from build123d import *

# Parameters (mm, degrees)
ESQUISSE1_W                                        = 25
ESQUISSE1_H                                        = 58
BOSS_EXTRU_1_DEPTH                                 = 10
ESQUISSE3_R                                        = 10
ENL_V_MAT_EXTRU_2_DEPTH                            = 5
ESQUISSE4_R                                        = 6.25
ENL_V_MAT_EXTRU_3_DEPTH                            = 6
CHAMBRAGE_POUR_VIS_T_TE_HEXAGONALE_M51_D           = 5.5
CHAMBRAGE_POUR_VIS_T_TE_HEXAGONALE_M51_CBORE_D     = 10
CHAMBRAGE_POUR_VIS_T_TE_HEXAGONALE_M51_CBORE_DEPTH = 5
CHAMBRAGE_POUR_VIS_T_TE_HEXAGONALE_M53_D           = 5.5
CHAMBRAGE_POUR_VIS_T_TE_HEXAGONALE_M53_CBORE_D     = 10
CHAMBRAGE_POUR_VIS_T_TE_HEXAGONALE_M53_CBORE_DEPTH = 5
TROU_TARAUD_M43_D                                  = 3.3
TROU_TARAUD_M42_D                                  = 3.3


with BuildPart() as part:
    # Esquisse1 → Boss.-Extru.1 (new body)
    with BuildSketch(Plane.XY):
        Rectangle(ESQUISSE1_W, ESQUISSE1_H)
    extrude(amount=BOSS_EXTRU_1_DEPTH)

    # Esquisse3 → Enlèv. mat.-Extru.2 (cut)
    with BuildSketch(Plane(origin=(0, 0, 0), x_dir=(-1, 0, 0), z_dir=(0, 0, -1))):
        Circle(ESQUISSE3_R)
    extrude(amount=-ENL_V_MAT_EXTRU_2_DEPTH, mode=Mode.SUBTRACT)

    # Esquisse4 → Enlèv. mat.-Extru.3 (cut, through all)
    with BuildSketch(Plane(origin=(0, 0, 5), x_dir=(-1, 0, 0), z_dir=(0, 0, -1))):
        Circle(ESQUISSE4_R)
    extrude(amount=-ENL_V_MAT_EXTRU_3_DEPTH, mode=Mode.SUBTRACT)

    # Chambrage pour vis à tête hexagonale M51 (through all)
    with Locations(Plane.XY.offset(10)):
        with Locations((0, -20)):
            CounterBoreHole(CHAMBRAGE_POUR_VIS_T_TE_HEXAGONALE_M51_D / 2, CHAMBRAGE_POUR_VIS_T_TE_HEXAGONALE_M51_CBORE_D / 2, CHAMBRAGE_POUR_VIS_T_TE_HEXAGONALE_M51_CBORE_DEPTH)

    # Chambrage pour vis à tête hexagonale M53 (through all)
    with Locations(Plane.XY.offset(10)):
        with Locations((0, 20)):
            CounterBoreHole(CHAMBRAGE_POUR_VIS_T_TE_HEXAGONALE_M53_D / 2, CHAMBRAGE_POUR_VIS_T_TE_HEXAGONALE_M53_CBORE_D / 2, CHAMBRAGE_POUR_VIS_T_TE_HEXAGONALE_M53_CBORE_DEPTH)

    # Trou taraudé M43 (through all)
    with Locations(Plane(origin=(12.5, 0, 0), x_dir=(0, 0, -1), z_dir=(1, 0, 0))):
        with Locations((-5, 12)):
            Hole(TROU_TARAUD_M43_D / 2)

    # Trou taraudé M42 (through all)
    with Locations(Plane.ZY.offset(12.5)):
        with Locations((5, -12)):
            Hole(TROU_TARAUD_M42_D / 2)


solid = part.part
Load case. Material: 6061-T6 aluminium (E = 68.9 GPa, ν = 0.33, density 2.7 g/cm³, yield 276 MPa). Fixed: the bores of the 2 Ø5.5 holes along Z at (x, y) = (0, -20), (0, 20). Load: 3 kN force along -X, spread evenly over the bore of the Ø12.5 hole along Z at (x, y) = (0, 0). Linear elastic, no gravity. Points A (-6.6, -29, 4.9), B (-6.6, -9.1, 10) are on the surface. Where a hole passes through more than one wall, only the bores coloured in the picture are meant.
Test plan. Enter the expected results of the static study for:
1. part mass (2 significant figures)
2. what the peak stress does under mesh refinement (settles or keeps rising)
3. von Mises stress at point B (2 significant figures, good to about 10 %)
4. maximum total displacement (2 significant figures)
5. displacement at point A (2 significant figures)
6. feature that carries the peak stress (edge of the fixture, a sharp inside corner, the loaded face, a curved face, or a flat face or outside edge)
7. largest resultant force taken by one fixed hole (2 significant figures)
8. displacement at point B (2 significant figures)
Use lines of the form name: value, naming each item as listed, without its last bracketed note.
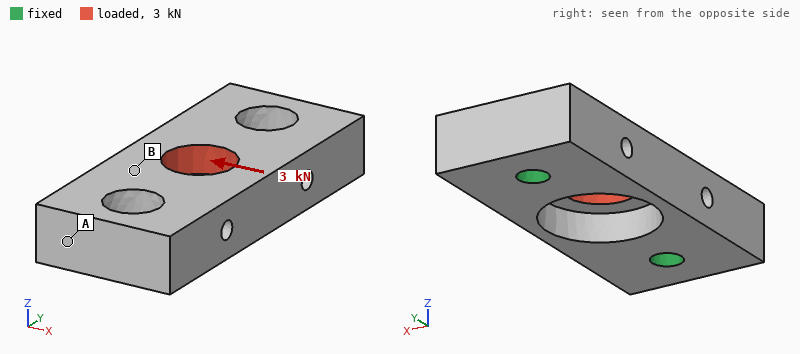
part mass: 29 g
what the peak stress does under mesh refinement: keeps rising
von Mises stress at point B: 21 MPa
maximum total displacement: 26 µm
displacement at point A: 4.6 µm
feature that carries the peak stress: edge of the fixture
largest resultant force taken by one fixed hole: 1.5 kN
displacement at point B: 18 µm
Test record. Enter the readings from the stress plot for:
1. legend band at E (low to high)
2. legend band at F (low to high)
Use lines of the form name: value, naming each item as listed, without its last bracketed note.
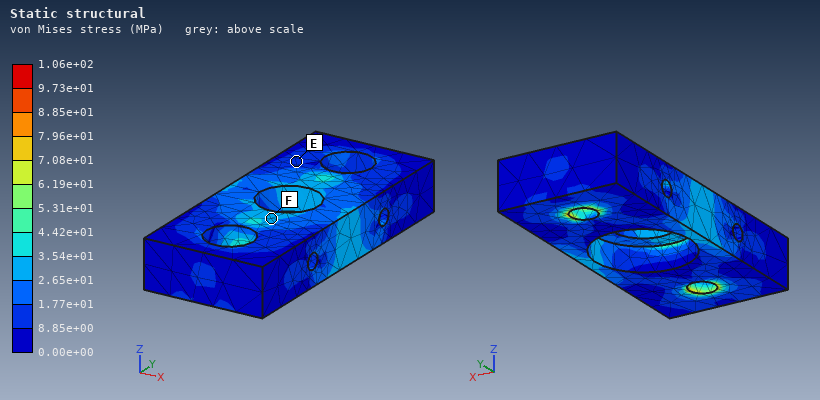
legend band at E: 8.85e+00 to 1.77e+01 MPa
legend band at F: 2.65e+01 to 3.54e+01 MPa
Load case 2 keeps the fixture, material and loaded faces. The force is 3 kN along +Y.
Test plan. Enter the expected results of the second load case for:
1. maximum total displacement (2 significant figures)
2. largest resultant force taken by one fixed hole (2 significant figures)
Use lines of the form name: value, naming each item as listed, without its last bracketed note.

maximum total displacement: 6.3 µm
largest resultant force taken by one fixed hole: 1.5 kN
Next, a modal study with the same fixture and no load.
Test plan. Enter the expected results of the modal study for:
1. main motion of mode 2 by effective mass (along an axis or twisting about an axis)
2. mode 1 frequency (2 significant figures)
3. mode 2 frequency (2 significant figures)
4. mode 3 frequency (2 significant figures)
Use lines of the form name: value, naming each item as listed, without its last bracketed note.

main motion of mode 2 by effective mass: along Z
mode 1 frequency: 13 kHz
mode 2 frequency: 18 kHz
mode 3 frequency: 20 kHz
